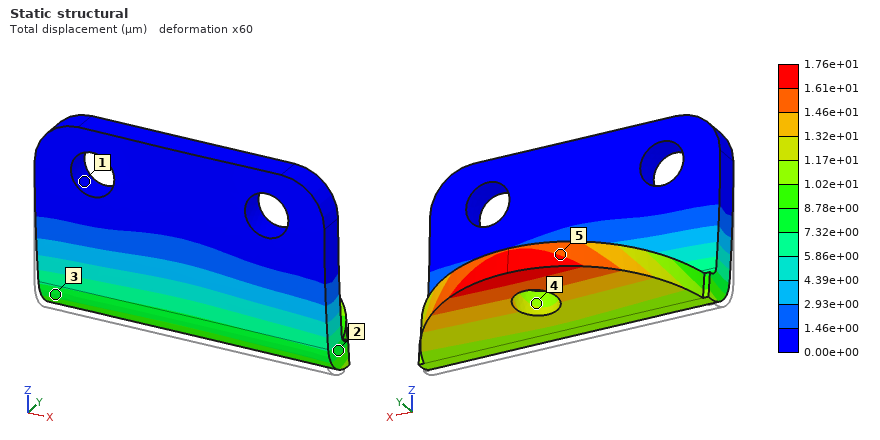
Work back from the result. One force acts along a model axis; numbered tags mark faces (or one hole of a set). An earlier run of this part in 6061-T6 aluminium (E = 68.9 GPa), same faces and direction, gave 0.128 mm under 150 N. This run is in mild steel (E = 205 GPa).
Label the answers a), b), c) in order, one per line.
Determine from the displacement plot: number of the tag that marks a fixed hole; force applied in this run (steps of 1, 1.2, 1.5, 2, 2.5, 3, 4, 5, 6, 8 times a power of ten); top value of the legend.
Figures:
a) 1
b) 60 N
c) 1.76e+01 µm
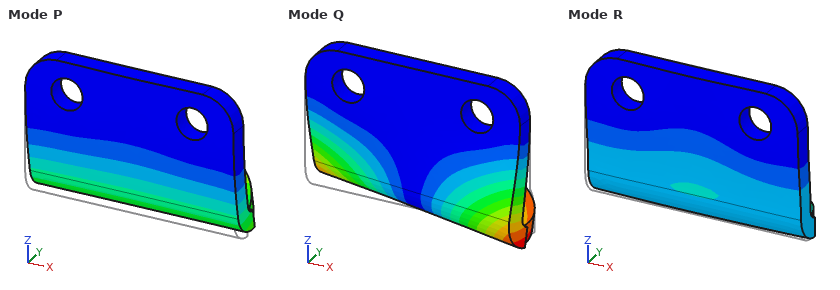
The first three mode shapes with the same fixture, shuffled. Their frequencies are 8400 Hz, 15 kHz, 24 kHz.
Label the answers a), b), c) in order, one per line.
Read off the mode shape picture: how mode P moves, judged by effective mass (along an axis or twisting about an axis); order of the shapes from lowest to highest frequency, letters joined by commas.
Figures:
a) along Y
b) P, Q, R
